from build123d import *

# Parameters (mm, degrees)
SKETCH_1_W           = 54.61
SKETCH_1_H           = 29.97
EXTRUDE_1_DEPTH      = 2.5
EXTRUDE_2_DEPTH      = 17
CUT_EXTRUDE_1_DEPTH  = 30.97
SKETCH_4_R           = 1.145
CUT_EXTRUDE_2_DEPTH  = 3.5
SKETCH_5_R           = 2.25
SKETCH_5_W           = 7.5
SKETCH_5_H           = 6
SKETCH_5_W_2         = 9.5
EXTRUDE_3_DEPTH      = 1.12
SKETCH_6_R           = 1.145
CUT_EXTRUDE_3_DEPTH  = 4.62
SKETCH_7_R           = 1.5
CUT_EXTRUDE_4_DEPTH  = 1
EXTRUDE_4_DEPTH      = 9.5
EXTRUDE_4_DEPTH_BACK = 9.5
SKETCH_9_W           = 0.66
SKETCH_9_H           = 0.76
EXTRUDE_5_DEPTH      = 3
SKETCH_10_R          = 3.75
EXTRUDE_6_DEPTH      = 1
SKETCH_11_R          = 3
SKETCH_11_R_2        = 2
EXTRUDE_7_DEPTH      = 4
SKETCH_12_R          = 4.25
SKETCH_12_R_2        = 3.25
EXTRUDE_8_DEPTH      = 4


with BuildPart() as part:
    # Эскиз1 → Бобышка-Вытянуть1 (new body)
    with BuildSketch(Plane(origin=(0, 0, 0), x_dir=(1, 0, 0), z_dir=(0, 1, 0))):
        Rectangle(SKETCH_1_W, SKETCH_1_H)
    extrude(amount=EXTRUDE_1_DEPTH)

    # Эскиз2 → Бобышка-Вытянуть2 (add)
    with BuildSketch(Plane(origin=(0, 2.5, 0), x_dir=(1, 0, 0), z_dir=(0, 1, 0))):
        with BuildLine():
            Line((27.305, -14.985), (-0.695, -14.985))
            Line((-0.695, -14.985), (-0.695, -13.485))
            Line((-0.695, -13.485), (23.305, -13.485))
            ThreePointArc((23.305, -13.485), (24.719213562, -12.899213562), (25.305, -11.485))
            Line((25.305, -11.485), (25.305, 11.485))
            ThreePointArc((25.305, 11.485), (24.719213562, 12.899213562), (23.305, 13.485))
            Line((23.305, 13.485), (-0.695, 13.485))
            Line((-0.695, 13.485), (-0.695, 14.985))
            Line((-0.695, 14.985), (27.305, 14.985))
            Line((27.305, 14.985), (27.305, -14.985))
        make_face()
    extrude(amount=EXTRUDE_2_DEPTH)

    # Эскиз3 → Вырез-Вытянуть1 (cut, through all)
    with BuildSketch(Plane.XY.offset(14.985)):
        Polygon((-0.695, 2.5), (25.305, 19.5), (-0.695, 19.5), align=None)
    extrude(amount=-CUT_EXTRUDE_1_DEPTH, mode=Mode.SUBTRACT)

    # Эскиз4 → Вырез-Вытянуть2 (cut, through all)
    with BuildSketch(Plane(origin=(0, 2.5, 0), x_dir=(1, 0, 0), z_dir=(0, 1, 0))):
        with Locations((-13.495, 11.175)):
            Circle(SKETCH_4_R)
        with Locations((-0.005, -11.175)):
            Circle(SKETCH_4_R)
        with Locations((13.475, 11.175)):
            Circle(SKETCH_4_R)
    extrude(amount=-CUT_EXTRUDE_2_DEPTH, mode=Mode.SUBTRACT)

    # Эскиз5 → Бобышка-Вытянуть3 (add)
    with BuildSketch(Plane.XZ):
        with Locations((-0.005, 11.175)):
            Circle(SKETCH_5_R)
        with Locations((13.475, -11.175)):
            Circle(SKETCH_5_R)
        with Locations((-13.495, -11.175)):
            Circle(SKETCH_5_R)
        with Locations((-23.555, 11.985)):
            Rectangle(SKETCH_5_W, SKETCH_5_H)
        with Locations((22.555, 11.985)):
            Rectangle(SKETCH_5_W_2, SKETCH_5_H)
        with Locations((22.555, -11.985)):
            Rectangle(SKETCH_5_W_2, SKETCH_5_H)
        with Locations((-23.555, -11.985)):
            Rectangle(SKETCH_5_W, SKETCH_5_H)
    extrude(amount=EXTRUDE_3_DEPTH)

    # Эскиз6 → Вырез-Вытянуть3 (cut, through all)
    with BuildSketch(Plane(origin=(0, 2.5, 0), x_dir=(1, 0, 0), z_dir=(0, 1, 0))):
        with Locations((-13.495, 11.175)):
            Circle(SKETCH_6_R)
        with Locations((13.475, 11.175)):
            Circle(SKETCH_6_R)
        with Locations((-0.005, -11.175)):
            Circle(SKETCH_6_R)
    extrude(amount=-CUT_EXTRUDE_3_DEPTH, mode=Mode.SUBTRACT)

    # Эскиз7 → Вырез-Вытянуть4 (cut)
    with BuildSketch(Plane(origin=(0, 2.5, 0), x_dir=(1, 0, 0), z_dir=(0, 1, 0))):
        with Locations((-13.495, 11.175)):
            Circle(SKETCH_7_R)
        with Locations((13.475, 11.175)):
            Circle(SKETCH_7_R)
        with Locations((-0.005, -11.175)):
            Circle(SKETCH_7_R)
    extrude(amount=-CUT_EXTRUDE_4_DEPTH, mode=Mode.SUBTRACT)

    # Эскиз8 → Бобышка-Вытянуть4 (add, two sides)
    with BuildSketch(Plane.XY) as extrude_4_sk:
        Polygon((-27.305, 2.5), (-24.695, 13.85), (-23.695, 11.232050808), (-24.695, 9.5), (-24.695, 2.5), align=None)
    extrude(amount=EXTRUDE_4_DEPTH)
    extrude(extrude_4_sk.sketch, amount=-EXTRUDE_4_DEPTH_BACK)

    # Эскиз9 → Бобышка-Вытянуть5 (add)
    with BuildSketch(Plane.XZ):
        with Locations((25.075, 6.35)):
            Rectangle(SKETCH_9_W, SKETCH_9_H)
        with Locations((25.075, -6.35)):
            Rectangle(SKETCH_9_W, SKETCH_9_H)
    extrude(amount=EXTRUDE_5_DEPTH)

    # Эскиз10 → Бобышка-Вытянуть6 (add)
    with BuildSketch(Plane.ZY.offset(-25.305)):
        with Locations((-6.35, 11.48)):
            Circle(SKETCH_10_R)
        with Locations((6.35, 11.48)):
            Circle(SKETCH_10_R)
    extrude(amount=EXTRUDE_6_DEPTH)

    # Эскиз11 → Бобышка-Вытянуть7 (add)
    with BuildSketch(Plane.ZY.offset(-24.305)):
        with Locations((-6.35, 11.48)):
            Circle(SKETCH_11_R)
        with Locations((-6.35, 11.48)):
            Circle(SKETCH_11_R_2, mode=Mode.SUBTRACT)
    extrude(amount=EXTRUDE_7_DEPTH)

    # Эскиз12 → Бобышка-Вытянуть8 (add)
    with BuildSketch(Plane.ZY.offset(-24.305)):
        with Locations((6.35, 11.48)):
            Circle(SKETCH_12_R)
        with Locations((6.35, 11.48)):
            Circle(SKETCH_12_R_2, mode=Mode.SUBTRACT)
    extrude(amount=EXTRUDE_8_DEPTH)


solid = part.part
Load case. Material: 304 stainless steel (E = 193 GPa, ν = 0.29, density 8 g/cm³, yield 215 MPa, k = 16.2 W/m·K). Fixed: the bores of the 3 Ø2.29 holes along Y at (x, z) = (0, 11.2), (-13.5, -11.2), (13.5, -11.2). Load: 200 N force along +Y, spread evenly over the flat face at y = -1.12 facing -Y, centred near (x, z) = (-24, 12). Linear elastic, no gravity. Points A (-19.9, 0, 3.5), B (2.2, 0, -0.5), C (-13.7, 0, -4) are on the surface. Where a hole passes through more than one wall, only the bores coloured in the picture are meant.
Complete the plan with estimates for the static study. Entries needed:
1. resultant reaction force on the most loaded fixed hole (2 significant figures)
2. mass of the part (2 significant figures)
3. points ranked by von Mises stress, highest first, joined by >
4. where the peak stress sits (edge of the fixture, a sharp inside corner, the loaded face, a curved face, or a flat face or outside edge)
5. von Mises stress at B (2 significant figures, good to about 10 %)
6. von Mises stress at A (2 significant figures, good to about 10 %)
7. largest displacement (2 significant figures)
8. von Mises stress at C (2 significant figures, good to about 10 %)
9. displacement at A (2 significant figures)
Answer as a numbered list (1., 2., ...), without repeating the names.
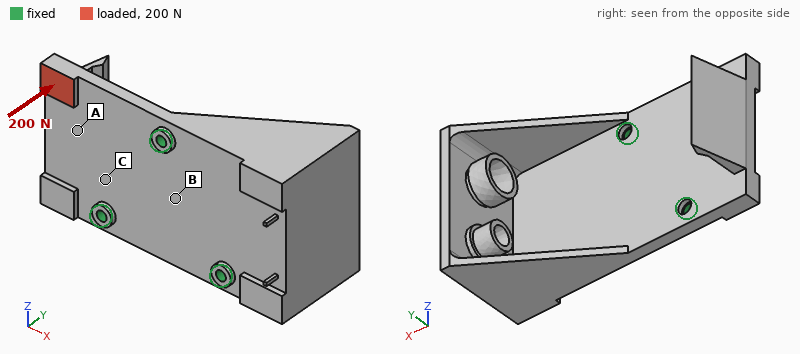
1. 190 N
2. 53 g
3. C > A > B
4. edge of the fixture
5. 19 MPa
6. 50 MPa
7. 0.13 mm
8. 79 MPa
9. 0.050 mm
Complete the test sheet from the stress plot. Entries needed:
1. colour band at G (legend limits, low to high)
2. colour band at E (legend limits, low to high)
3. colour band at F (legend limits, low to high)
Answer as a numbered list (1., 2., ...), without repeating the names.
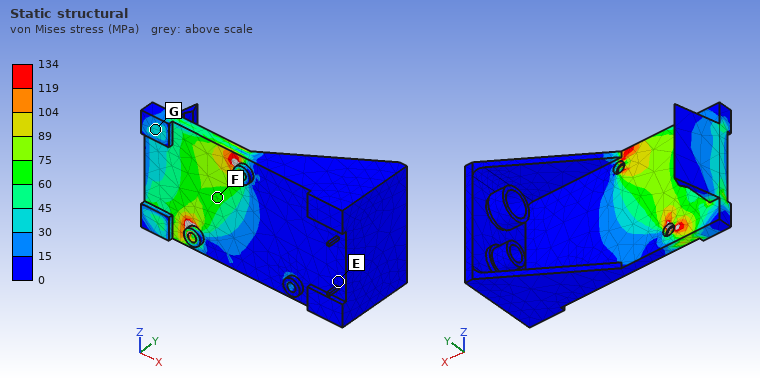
1. 30 to 45 MPa
2. 0 to 15 MPa
3. 60 to 75 MPa
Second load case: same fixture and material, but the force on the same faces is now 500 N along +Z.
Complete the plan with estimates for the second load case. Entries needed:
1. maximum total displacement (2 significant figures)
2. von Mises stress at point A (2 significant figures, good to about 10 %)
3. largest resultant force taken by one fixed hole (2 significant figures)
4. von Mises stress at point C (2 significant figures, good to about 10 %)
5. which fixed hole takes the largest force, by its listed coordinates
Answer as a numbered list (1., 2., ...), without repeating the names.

1. 31 µm
2. 36 MPa
3. 490 N
4. 29 MPa
5. (-13.5, -11.2)
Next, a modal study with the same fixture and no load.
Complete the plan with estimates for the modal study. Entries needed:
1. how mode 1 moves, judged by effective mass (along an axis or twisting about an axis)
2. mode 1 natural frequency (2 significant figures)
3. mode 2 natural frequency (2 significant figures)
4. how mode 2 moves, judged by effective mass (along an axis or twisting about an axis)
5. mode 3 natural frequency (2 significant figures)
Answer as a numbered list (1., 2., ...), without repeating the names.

1. along Y
2. 2500 Hz
3. 3300 Hz
4. along Y
5. 5800 Hz
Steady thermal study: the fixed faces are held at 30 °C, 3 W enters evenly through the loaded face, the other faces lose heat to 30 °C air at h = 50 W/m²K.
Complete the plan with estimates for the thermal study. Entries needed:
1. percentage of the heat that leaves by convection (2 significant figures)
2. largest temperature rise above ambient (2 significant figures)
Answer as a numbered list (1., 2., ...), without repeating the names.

1. 60 %
2. 62 K
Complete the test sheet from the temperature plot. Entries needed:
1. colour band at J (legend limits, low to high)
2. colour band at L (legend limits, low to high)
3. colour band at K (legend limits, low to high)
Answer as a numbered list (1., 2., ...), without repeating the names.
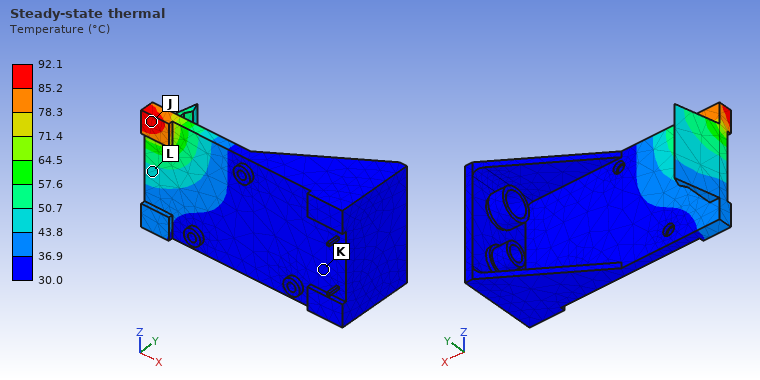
1. 85.2 to 92.1 °C
2. 43.8 to 50.7 °C
3. 30.0 to 36.9 °C
